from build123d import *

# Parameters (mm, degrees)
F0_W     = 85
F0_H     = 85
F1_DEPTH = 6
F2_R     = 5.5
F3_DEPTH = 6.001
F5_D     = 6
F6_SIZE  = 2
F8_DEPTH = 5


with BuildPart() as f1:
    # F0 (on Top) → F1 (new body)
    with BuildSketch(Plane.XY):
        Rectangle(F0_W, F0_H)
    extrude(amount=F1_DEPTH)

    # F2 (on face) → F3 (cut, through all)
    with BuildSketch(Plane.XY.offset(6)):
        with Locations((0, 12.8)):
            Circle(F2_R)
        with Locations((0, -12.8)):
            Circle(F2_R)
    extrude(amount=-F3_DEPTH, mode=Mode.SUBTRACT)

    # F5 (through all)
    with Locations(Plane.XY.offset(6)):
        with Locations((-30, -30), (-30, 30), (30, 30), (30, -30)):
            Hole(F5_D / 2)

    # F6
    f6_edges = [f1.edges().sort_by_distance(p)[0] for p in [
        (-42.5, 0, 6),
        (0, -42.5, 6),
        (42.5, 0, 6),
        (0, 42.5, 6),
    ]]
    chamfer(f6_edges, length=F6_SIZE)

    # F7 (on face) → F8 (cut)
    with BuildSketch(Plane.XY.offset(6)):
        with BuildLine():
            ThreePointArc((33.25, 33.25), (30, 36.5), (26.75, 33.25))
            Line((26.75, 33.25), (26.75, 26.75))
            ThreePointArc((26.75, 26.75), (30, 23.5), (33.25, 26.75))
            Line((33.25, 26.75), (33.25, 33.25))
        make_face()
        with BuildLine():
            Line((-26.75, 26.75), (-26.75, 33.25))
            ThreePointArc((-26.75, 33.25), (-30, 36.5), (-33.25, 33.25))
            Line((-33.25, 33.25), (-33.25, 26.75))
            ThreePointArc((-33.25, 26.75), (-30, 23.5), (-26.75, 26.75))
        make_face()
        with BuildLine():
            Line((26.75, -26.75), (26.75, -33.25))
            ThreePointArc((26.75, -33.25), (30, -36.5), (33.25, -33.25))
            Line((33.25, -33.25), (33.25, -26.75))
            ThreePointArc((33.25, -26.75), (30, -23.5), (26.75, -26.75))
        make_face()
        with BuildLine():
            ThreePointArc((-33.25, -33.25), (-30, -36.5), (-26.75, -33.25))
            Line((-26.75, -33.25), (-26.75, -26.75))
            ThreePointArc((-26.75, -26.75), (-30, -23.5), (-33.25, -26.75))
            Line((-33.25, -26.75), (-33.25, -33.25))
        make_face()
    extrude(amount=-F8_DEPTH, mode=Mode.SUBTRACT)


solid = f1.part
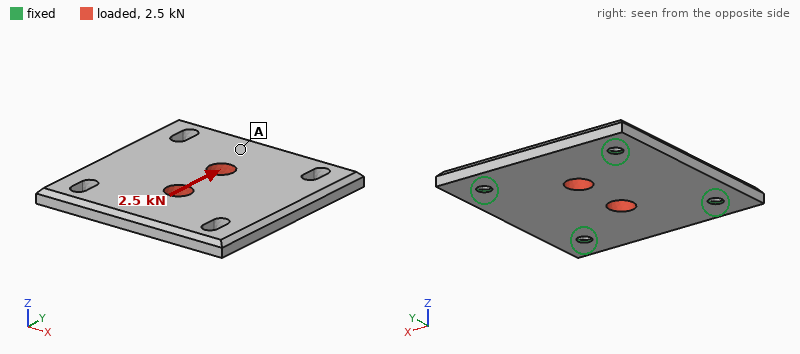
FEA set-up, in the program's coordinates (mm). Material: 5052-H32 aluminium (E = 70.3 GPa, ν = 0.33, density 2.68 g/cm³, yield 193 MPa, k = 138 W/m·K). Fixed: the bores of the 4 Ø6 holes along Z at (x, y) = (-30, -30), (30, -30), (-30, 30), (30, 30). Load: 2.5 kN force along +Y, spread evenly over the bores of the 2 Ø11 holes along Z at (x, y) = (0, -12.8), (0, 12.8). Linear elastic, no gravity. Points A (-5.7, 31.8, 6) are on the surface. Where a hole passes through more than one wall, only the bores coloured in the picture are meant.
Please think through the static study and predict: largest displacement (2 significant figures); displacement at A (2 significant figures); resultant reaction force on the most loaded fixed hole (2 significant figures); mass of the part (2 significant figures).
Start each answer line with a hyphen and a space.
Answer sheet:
- 6.7 µm
- 5.2 µm
- 640 N
- 110 g
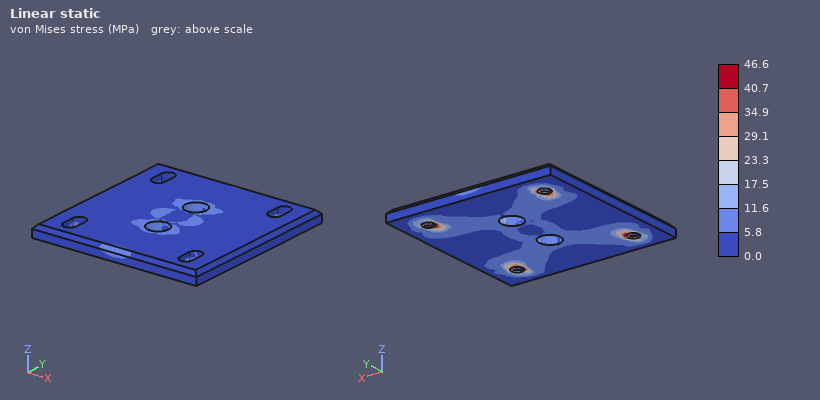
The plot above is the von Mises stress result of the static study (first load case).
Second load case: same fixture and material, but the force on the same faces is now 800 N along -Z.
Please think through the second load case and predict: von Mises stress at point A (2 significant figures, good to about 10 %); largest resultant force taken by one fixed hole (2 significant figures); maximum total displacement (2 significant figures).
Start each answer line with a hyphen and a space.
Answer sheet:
- 13 MPa
- 560 N
- 39 µm
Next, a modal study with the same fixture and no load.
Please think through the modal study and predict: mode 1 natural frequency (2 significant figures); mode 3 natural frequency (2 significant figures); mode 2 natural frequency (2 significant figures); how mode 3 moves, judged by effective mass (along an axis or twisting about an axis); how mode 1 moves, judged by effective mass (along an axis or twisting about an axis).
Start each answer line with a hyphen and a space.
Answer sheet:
- 4500 Hz
- 6300 Hz
- 5900 Hz
- twisting about Y
- along Z
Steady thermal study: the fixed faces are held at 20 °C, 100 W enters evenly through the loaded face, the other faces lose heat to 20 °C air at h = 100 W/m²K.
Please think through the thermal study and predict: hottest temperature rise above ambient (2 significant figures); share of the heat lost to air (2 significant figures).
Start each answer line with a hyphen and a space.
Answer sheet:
- 42 K
- 31 %
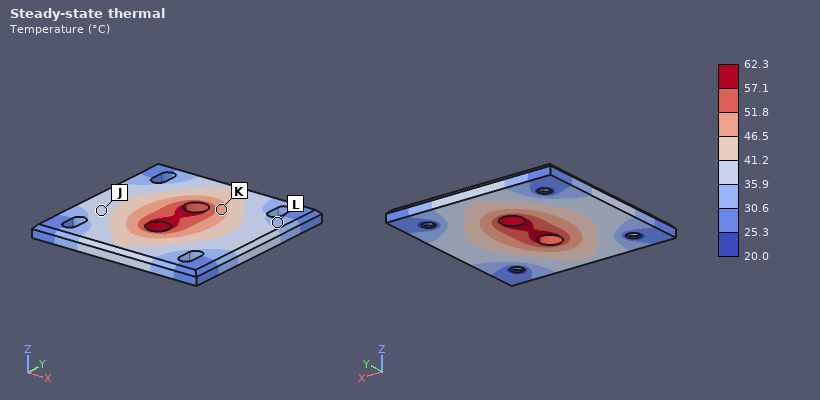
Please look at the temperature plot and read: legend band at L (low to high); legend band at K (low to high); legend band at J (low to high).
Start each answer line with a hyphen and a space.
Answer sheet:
- 30.6 to 35.9 °C
- 46.5 to 51.8 °C
- 35.9 to 41.2 °C
